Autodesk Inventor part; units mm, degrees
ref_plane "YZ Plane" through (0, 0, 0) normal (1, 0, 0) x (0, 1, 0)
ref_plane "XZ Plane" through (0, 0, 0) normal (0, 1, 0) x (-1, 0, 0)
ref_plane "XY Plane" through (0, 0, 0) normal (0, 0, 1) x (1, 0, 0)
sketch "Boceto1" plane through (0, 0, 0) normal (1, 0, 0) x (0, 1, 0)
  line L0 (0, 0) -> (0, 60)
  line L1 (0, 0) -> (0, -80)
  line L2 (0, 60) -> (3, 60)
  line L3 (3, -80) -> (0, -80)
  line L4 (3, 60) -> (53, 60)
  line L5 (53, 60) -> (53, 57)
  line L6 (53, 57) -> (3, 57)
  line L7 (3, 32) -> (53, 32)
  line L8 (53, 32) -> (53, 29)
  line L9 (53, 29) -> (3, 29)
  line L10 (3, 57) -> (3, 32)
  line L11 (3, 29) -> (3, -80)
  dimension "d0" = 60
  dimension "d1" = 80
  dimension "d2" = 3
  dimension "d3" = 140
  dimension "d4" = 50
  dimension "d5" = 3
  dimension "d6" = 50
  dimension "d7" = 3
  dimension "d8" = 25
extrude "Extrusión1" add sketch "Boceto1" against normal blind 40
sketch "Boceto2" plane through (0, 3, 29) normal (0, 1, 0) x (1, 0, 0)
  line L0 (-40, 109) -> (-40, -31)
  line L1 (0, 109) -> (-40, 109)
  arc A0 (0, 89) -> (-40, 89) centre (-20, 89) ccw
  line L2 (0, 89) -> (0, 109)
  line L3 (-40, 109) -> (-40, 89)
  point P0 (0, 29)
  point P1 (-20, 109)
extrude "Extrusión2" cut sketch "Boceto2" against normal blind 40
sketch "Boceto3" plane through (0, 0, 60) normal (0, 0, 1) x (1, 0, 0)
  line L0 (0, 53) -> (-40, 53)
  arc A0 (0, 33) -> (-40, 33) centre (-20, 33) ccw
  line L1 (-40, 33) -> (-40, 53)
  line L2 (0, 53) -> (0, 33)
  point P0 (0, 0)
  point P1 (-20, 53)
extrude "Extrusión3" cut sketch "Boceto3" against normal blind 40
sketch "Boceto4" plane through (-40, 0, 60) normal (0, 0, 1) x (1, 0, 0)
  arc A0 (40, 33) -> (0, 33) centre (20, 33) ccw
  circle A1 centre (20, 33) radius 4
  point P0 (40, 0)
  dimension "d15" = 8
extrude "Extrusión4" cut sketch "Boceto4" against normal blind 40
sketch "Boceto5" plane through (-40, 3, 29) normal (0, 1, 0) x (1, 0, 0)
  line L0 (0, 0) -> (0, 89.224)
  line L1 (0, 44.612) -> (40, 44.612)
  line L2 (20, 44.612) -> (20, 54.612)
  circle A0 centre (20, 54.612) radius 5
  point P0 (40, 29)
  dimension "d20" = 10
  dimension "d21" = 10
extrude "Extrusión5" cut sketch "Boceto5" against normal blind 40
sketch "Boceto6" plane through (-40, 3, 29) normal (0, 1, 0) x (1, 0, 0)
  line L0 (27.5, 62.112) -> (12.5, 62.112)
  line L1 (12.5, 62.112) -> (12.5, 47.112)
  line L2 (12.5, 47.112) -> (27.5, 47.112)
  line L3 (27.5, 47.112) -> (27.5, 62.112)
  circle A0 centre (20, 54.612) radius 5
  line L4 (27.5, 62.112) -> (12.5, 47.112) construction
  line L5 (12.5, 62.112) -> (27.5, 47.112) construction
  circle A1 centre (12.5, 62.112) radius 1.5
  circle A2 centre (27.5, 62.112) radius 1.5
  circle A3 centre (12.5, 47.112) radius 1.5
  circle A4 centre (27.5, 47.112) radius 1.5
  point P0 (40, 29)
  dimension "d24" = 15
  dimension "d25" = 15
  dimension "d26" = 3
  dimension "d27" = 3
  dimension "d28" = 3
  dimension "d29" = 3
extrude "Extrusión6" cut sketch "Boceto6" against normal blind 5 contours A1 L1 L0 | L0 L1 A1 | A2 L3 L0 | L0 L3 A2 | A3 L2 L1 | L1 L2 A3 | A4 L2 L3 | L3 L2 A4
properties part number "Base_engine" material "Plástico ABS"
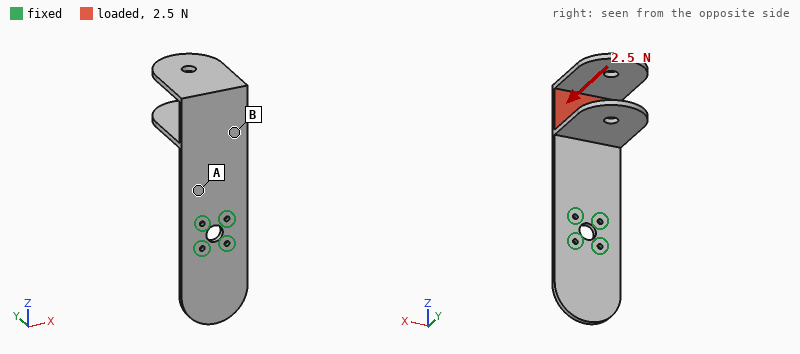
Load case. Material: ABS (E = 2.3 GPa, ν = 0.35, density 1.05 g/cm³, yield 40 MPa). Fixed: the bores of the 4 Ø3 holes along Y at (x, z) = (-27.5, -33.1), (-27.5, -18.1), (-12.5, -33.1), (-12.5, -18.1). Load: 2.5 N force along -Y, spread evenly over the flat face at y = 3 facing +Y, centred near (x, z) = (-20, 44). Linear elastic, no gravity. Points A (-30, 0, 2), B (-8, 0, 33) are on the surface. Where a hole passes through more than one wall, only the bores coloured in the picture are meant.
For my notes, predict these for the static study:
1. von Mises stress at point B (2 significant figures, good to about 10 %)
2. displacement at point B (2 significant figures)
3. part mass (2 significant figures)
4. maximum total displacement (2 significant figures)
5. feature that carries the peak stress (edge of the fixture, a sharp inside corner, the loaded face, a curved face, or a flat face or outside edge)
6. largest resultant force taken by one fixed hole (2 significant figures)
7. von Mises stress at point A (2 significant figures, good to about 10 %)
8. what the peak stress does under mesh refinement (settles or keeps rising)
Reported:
0.40 MPa
0.70 mm
28 g
1.8 mm
edge of the fixture
2.7 N
1.6 MPa
keeps rising
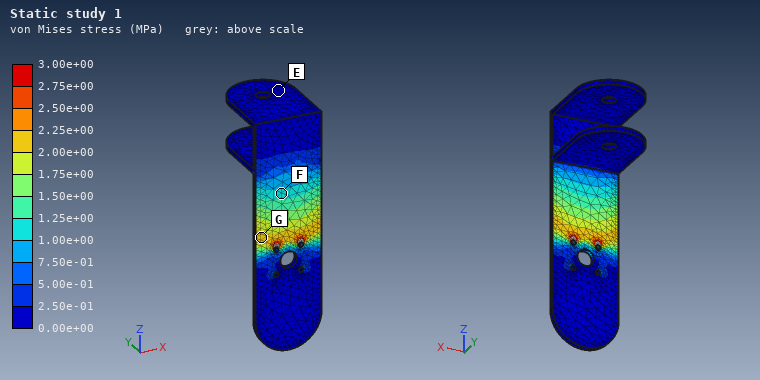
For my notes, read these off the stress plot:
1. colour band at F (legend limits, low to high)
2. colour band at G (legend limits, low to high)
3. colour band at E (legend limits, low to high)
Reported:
1.00e+00 to 1.25e+00 MPa
2.00e+00 to 2.25e+00 MPa
0.00e+00 to 2.50e-01 MPa
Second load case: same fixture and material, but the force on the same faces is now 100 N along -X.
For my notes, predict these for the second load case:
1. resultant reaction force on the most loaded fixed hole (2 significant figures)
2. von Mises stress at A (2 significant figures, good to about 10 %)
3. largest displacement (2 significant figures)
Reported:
220 N
2.8 MPa
1.7 mm
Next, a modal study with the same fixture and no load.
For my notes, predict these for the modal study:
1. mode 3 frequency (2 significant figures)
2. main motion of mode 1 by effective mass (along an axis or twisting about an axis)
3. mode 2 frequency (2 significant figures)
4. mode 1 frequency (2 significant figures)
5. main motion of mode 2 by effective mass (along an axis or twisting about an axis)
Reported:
200 Hz
along Y
130 Hz
54 Hz
along X
